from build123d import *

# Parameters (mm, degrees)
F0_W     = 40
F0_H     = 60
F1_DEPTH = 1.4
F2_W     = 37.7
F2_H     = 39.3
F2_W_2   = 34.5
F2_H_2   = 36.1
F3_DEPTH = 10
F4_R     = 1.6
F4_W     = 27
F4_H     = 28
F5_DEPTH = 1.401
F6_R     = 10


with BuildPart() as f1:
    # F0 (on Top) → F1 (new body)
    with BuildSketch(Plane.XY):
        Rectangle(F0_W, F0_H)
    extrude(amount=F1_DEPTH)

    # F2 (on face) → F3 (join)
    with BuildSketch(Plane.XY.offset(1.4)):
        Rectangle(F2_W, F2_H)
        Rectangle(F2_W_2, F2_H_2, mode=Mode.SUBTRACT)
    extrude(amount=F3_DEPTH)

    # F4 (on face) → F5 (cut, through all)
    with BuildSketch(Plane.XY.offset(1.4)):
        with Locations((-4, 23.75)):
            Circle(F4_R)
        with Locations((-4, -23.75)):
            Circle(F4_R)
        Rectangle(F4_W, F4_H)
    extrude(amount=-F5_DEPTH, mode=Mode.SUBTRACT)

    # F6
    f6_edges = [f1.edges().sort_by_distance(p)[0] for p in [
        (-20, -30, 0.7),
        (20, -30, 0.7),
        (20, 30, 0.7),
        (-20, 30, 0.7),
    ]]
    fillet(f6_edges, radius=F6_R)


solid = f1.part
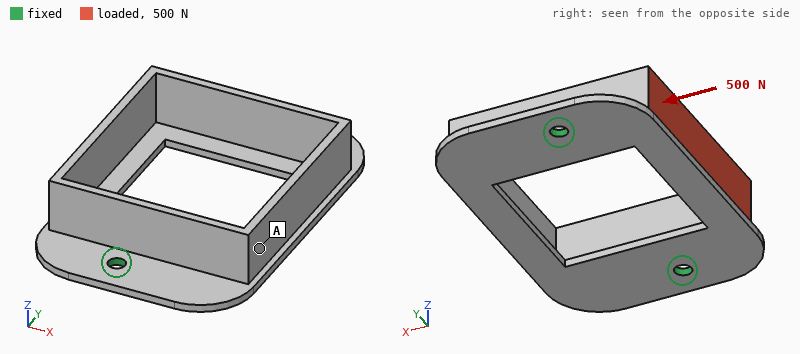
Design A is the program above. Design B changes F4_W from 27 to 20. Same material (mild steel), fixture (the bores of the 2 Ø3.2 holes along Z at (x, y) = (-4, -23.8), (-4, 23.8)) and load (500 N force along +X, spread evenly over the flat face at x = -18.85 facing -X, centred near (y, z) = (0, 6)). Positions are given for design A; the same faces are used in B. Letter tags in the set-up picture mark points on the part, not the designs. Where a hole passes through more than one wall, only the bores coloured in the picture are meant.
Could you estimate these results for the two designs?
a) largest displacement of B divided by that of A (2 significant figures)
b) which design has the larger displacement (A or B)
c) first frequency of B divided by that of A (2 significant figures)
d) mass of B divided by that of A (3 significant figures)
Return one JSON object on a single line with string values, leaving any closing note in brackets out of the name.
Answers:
{"largest displacement of B divided by that of A": "0.92", "which design has the larger displacement": "A", "first frequency of B divided by that of A": "0.98", "mass of B divided by that of A": "1.06"}
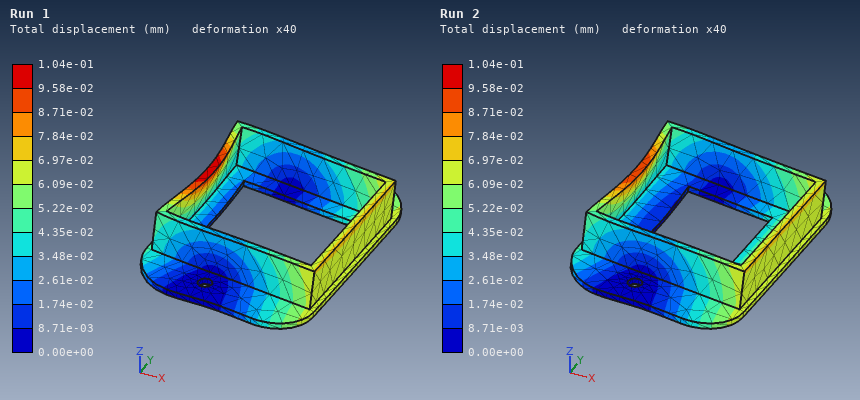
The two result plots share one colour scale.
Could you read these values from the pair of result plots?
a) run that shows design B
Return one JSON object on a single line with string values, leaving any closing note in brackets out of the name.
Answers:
{"run that shows design B": "Run 2"}
